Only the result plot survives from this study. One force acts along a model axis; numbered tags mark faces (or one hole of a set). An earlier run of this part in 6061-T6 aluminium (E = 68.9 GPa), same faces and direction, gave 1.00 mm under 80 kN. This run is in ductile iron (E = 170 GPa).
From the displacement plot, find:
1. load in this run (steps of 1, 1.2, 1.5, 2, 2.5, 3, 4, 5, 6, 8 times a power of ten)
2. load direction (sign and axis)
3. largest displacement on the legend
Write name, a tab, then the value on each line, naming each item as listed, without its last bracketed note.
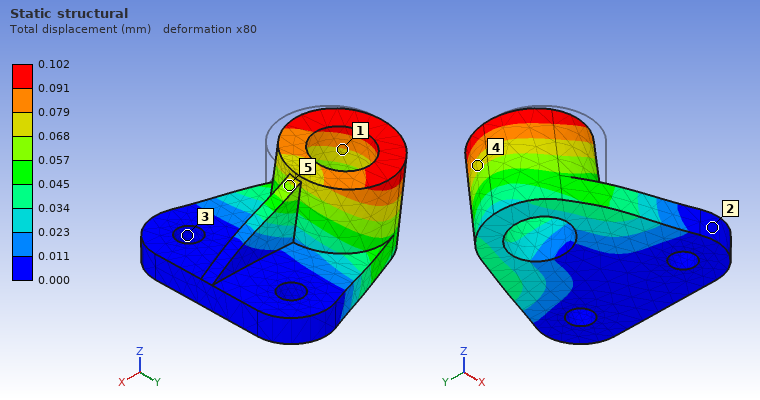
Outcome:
load in this run	20 kN
load direction	+Y
largest displacement on the legend	0.102 mm
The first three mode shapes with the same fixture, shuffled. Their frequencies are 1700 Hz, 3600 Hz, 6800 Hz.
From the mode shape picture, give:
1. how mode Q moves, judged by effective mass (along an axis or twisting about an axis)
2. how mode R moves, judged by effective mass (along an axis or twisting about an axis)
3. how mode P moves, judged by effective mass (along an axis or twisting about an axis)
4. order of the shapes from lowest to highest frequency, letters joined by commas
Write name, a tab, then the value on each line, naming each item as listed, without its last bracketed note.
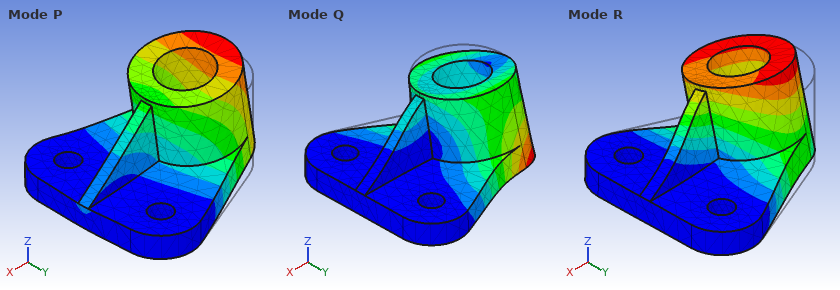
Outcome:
how mode Q moves, judged by effective mass	along Y
how mode R moves, judged by effective mass	along Y
how mode P moves, judged by effective mass	along Z
order of the shapes from lowest to highest frequency, letters joined by commas	P, R, Q
